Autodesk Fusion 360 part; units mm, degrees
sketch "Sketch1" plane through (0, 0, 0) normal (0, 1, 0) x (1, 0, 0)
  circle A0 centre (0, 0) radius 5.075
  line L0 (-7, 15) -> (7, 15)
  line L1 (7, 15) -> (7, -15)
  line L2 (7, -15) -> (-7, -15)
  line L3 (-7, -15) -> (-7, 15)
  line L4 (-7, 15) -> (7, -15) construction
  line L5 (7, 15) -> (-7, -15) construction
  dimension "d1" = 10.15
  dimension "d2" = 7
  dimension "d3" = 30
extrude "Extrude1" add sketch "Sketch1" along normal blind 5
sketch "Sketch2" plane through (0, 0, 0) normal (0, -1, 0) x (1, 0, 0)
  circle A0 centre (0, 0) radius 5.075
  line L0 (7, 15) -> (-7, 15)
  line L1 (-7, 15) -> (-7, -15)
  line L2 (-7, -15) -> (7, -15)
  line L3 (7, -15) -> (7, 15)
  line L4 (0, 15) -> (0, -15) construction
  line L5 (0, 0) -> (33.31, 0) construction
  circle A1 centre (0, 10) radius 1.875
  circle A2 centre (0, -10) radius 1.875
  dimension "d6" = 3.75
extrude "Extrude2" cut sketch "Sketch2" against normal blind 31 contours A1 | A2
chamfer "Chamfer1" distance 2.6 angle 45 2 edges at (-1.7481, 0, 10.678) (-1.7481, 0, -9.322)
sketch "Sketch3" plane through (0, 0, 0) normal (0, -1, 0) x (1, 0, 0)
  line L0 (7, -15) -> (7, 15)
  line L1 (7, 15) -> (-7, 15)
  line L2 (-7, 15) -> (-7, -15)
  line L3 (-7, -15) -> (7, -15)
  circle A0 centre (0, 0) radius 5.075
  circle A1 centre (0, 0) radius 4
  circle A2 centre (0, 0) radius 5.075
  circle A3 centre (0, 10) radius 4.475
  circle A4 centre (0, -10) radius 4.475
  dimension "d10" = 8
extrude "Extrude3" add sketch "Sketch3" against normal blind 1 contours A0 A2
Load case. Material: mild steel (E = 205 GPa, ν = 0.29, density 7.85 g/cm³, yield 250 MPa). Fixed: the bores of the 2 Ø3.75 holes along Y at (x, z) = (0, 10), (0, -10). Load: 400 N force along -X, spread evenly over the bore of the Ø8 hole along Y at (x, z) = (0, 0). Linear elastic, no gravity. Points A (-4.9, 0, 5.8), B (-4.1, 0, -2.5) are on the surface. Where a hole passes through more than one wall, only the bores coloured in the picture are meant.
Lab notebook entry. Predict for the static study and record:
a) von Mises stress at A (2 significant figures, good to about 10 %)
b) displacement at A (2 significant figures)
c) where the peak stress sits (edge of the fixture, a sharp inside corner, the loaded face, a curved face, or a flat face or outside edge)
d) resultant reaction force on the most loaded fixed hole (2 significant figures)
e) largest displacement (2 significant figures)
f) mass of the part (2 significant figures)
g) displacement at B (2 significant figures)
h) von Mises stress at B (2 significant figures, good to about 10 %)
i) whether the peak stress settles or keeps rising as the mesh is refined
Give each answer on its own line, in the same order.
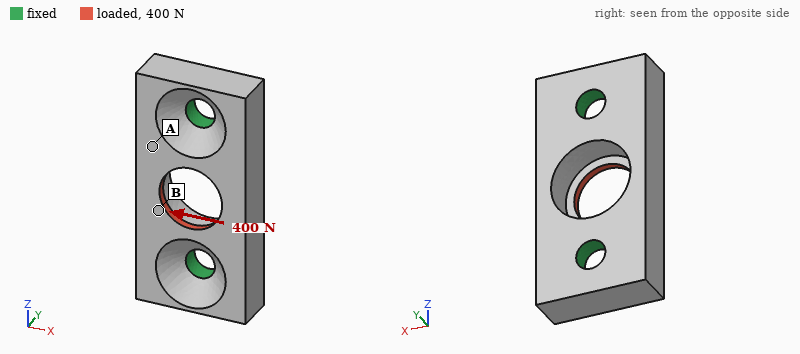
9.4 MPa
1.3 µm
edge of the fixture
200 N
2.3 µm
12 g
1.7 µm
20 MPa
keeps rising
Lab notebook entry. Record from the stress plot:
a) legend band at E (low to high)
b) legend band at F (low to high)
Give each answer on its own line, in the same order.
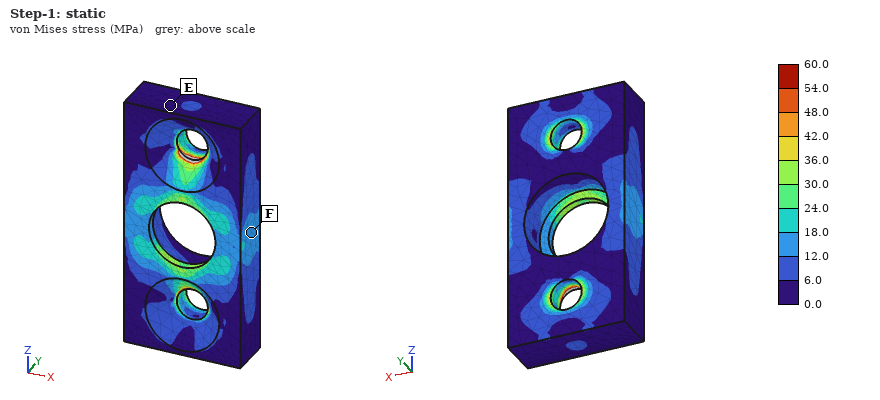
0.0 to 6.0 MPa
12.0 to 18.0 MPa
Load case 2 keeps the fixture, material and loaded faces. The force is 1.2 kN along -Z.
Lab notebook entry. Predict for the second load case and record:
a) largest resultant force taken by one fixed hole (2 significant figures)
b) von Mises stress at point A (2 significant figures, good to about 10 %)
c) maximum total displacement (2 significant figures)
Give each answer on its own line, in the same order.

620 N
19 MPa
2.7 µm
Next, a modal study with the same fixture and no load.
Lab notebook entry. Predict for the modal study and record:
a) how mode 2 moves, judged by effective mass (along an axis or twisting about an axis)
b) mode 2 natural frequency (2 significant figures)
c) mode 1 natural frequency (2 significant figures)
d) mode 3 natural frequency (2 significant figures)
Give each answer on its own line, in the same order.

along Y
39 kHz
30 kHz
42 kHz
